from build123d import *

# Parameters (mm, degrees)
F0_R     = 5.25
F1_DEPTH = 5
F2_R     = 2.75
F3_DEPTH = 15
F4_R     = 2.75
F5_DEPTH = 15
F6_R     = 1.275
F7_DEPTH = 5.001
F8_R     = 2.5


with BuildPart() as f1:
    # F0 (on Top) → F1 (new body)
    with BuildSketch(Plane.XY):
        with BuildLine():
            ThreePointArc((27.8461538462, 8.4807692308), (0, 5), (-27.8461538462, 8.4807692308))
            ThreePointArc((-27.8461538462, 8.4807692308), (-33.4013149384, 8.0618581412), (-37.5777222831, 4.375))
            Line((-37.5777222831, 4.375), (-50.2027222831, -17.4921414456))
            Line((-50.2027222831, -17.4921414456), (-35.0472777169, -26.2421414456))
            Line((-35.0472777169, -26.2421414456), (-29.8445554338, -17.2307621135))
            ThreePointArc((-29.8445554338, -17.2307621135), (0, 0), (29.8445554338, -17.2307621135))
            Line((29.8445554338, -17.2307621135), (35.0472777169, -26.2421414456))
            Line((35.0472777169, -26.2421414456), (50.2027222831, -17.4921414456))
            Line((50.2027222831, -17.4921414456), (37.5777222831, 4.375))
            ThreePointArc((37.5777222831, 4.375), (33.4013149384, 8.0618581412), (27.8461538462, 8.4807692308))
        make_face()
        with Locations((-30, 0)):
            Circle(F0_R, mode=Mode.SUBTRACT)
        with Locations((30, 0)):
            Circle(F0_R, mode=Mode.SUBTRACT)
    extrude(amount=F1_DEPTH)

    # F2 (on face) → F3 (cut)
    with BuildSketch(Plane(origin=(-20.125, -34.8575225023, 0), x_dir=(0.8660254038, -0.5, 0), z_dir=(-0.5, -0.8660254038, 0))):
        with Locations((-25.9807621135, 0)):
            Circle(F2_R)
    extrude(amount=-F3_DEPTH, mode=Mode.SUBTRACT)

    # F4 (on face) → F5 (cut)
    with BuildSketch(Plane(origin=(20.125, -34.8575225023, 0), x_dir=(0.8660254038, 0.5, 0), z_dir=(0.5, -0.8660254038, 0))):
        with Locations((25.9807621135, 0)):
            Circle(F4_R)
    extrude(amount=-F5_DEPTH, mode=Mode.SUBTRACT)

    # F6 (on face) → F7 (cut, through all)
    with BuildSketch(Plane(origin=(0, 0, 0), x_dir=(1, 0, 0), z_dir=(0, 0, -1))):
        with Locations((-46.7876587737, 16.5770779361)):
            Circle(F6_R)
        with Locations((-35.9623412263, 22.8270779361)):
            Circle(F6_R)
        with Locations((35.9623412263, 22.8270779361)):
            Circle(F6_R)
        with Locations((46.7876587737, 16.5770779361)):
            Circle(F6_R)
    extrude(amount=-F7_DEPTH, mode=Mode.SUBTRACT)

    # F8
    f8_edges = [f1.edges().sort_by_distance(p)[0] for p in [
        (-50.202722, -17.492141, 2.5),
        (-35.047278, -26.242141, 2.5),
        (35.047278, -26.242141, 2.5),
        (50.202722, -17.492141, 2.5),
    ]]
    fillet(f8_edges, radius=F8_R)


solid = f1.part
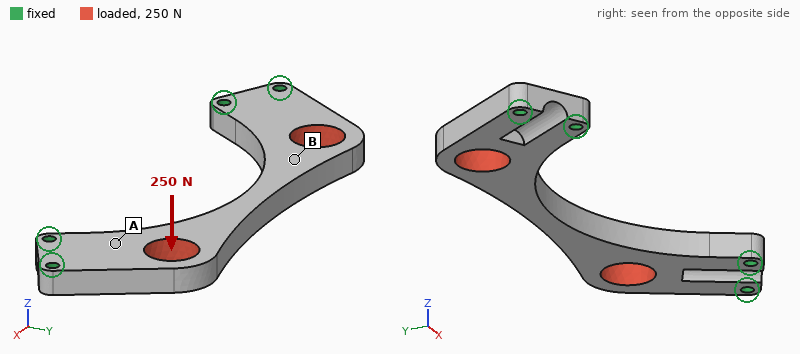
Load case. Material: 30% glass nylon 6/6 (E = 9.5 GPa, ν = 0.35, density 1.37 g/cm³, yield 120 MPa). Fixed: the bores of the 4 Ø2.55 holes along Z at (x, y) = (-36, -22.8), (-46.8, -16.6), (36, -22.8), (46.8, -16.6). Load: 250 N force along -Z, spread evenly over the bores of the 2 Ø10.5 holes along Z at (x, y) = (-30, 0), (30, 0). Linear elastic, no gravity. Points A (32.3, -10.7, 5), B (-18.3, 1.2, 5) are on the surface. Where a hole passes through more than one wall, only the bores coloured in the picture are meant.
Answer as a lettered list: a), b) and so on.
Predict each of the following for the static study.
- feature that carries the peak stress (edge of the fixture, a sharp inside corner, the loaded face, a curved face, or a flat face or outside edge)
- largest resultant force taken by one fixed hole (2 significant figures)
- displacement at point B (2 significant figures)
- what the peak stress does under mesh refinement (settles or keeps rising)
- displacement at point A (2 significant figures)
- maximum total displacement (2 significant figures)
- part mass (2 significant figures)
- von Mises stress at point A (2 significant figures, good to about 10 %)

a) edge of the fixture
b) 81 N
c) 0.45 mm
d) keeps rising
e) 0.13 mm
f) 0.58 mm
g) 8.5 g
h) 17 MPa
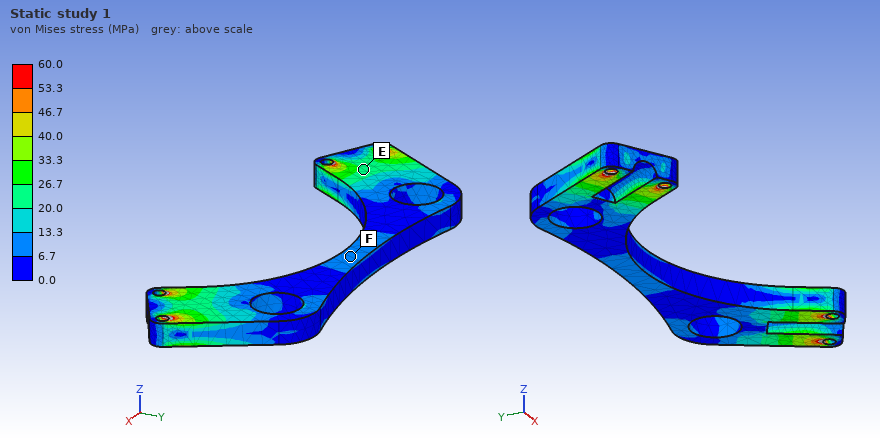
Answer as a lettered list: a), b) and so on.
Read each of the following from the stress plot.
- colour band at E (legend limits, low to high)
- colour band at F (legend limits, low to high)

a) 20.0 to 26.7 MPa
b) 6.7 to 13.3 MPa
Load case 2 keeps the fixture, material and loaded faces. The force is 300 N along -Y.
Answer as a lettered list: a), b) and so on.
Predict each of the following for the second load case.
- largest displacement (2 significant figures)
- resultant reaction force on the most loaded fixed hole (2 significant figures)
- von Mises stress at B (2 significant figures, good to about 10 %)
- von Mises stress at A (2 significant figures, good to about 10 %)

a) 15 µm
b) 130 N
c) 1.0 MPa
d) 1.5 MPa
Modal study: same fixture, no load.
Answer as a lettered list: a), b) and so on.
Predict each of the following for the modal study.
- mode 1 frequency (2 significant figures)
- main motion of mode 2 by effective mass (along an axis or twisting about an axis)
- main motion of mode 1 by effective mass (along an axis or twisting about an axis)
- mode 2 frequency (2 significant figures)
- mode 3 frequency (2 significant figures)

a) 1400 Hz
b) twisting about Y
c) along Z
d) 2800 Hz
e) 4500 Hz
